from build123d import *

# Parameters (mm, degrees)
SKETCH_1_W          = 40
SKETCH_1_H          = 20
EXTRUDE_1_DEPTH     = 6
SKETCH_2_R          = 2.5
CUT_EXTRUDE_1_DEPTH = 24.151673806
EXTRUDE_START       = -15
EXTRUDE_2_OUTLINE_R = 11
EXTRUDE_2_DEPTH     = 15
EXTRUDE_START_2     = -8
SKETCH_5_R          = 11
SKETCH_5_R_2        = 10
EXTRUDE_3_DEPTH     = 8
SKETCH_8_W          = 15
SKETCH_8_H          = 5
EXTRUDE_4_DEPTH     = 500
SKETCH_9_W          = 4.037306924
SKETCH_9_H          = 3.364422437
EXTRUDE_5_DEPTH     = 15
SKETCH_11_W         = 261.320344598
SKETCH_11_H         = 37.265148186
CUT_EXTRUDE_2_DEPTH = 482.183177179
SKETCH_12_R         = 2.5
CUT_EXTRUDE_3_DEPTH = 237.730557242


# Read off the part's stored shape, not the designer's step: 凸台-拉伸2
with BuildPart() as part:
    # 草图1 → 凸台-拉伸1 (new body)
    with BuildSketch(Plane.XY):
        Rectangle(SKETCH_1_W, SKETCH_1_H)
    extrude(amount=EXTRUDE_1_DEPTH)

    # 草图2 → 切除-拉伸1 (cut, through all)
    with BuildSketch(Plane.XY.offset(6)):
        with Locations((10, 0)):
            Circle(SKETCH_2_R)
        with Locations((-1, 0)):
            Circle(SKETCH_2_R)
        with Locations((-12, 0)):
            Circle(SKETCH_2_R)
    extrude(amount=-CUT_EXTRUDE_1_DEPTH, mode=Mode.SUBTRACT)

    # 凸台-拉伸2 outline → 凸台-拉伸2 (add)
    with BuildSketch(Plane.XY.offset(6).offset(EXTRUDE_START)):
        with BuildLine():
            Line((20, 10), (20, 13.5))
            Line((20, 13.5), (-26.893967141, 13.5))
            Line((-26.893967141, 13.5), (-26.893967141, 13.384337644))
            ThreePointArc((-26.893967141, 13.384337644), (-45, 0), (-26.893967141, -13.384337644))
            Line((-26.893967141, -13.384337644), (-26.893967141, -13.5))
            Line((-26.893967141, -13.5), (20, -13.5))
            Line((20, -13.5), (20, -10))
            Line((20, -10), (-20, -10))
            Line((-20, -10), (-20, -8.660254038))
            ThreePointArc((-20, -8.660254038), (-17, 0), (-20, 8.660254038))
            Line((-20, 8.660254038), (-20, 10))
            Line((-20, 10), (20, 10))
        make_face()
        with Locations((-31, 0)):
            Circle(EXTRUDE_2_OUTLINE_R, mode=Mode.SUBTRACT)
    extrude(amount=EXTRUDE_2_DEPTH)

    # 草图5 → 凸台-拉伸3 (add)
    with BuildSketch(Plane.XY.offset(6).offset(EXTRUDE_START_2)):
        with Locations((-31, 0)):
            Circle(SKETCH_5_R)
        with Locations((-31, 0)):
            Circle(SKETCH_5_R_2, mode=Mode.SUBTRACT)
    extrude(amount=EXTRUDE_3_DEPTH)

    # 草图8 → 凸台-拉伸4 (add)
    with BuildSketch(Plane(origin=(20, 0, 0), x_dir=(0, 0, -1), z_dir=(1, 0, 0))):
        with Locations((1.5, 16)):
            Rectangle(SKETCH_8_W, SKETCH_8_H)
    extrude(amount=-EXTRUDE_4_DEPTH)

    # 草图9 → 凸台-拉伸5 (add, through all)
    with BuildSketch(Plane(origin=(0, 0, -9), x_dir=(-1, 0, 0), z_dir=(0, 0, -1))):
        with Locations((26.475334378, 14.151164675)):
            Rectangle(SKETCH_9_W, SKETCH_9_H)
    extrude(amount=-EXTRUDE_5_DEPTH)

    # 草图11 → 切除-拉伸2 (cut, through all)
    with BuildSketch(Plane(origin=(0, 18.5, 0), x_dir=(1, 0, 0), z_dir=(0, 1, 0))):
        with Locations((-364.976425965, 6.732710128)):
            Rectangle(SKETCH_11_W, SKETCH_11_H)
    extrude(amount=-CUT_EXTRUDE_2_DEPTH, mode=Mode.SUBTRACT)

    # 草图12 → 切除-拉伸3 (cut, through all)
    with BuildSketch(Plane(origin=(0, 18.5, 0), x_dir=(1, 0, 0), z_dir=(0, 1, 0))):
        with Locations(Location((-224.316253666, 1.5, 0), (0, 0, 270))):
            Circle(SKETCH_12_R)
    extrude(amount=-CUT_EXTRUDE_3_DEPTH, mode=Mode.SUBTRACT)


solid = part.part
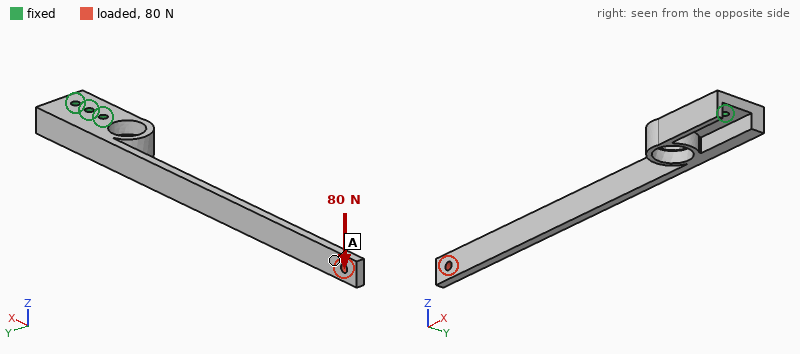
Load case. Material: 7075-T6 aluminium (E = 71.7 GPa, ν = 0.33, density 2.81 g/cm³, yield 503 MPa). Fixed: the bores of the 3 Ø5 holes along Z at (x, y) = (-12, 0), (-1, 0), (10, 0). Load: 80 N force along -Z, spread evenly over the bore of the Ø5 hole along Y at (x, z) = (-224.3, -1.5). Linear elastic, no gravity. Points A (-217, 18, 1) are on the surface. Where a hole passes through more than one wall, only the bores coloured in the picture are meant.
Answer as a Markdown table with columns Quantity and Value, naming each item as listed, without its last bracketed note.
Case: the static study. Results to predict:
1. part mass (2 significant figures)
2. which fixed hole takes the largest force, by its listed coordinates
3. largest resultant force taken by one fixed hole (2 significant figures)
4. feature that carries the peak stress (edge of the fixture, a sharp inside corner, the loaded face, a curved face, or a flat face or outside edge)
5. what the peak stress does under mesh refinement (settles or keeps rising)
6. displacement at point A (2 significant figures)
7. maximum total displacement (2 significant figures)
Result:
| Quantity | Value |
|---|---|
| part mass | 89 g |
| which fixed hole takes the largest force, by its listed coordinates | (-12, 0) |
| largest resultant force taken by one fixed hole | 720 N |
| feature that carries the peak stress | edge of the fixture |
| what the peak stress does under mesh refinement | keeps rising |
| displacement at point A | 2.2 mm |
| maximum total displacement | 2.5 mm |
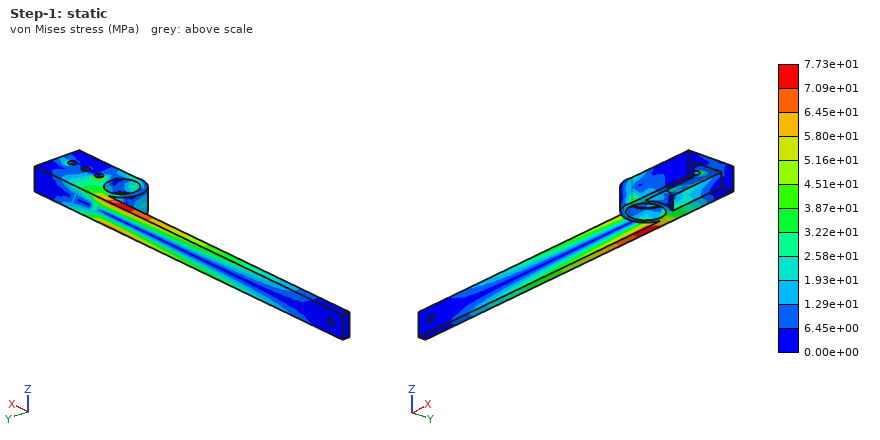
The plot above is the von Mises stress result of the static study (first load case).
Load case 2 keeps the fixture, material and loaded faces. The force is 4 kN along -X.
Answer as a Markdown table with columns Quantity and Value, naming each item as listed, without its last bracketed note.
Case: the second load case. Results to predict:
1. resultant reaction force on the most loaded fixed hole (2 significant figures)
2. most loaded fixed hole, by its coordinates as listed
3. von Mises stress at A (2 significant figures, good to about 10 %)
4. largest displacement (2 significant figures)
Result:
| Quantity | Value |
|---|---|
| resultant reaction force on the most loaded fixed hole | 3.0 kN |
| most loaded fixed hole, by its coordinates as listed | (-12, 0) |
| von Mises stress at A | 57 MPa |
| largest displacement | 0.58 mm |
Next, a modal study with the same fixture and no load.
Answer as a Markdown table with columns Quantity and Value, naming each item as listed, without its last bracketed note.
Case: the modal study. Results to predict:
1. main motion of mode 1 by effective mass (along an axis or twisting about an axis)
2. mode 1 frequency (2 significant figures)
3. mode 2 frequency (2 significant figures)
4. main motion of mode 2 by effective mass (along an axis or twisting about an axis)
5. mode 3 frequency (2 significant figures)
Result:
| Quantity | Value |
|---|---|
| main motion of mode 1 by effective mass | along Y |
| mode 1 frequency | 100 Hz |
| mode 2 frequency | 260 Hz |
| main motion of mode 2 by effective mass | along Z |
| mode 3 frequency | 620 Hz |
